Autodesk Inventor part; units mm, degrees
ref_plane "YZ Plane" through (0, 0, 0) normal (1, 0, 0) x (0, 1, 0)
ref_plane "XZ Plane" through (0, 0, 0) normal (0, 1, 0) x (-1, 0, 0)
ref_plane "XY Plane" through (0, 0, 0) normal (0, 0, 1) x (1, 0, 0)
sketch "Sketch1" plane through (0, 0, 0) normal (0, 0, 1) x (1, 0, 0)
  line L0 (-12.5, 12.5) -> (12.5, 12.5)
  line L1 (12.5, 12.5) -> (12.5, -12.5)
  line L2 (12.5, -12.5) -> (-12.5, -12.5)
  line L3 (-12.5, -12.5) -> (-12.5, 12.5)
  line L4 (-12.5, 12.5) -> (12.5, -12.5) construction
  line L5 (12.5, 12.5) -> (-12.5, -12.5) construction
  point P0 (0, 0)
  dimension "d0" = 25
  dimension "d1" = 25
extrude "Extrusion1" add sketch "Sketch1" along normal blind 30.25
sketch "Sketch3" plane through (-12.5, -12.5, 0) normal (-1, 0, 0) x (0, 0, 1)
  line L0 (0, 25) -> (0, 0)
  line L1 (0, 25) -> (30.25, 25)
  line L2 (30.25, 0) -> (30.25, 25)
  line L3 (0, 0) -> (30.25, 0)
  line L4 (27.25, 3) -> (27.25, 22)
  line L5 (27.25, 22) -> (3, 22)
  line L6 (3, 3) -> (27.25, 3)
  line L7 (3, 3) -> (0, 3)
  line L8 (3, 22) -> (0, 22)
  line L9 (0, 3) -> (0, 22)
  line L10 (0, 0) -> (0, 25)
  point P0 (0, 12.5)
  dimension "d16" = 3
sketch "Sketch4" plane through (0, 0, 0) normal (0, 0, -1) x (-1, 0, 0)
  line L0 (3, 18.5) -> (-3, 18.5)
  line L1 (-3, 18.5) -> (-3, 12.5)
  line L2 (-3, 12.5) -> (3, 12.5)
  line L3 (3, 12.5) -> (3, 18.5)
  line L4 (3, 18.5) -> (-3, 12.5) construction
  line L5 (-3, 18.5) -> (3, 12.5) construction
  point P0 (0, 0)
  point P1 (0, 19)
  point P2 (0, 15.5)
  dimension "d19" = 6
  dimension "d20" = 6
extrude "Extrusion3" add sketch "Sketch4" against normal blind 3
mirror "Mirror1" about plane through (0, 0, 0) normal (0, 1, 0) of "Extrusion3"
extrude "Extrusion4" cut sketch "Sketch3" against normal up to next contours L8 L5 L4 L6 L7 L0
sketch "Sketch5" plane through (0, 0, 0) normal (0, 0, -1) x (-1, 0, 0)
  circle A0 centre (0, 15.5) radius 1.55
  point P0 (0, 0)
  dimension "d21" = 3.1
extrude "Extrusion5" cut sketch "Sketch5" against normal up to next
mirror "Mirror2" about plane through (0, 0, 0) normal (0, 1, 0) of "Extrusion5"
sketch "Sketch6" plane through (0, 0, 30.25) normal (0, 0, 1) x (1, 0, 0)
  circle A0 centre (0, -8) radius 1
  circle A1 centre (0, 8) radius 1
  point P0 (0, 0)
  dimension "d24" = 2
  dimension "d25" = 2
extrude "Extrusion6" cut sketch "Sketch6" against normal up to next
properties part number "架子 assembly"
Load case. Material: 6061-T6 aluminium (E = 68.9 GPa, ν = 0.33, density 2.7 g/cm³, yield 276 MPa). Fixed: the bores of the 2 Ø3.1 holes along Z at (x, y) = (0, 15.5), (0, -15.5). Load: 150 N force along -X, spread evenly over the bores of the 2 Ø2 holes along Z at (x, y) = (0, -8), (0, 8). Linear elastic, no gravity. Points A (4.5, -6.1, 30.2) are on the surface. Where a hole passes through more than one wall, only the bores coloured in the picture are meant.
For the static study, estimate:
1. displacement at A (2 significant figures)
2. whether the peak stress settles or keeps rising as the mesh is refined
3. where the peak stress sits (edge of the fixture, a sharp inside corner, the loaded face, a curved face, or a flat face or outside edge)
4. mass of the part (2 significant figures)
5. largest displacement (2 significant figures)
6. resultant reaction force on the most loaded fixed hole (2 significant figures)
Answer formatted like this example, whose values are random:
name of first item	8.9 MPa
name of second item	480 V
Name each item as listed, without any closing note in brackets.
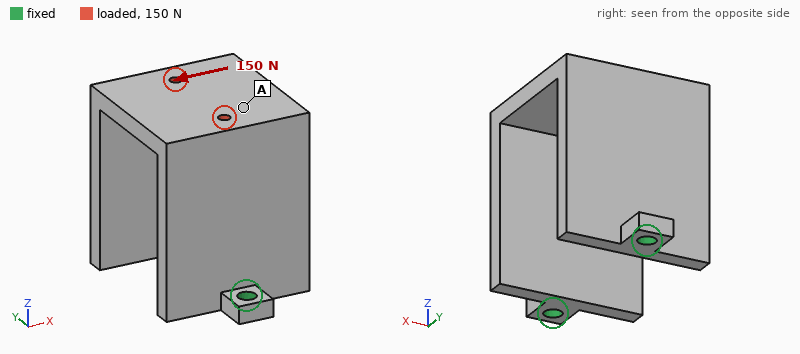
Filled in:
displacement at A	0.15 mm
whether the peak stress settles or keeps rising as the mesh is refined	keeps rising
where the peak stress sits	edge of the fixture
mass of the part	17 g
largest displacement	0.16 mm
resultant reaction force on the most loaded fixed hole	75 N
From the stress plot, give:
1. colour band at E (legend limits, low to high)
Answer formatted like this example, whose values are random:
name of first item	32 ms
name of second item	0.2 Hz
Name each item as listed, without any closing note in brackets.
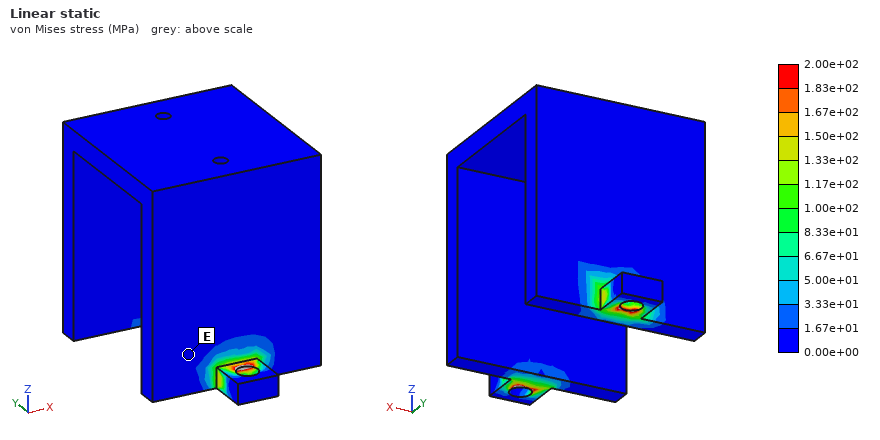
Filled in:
colour band at E	0.00e+00 to 1.67e+01 MPa
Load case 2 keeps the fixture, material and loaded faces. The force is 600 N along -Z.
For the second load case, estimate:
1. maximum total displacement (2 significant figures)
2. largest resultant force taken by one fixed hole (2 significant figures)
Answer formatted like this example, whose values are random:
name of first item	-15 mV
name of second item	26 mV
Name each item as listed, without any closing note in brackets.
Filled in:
maximum total displacement	12 µm
largest resultant force taken by one fixed hole	300 N
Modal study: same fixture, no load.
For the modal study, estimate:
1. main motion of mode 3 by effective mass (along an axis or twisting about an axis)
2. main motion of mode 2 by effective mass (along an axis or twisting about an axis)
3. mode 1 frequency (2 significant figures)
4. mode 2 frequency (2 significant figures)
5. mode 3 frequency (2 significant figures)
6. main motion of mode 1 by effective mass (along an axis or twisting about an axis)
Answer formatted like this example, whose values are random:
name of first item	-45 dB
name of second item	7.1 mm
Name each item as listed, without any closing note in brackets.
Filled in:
main motion of mode 3 by effective mass	twisting about Z
main motion of mode 2 by effective mass	along Y
mode 1 frequency	1700 Hz
mode 2 frequency	2500 Hz
mode 3 frequency	3800 Hz
main motion of mode 1 by effective mass	along X
